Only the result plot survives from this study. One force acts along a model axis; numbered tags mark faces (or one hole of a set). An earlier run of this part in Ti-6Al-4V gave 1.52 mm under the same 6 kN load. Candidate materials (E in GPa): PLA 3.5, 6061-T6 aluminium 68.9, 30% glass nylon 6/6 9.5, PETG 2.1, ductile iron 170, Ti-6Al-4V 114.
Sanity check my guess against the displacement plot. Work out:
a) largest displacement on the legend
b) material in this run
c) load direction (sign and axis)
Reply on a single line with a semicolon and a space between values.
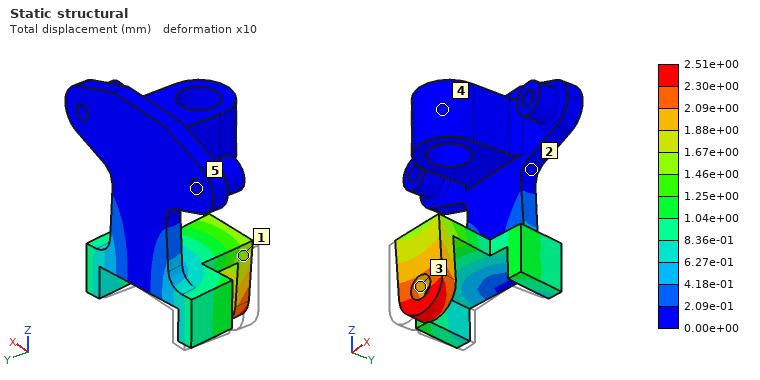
2.51e+00 mm; 6061-T6 aluminium; +X
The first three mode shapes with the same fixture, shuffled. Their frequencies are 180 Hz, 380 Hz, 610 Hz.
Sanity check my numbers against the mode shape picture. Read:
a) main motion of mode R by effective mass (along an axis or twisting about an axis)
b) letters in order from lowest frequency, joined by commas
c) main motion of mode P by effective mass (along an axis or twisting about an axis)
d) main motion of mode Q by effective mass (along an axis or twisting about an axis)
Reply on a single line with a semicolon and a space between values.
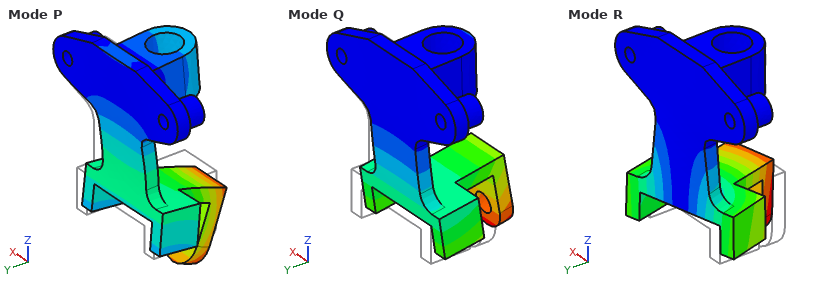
along X; Q, R, P; along Y; along Y
